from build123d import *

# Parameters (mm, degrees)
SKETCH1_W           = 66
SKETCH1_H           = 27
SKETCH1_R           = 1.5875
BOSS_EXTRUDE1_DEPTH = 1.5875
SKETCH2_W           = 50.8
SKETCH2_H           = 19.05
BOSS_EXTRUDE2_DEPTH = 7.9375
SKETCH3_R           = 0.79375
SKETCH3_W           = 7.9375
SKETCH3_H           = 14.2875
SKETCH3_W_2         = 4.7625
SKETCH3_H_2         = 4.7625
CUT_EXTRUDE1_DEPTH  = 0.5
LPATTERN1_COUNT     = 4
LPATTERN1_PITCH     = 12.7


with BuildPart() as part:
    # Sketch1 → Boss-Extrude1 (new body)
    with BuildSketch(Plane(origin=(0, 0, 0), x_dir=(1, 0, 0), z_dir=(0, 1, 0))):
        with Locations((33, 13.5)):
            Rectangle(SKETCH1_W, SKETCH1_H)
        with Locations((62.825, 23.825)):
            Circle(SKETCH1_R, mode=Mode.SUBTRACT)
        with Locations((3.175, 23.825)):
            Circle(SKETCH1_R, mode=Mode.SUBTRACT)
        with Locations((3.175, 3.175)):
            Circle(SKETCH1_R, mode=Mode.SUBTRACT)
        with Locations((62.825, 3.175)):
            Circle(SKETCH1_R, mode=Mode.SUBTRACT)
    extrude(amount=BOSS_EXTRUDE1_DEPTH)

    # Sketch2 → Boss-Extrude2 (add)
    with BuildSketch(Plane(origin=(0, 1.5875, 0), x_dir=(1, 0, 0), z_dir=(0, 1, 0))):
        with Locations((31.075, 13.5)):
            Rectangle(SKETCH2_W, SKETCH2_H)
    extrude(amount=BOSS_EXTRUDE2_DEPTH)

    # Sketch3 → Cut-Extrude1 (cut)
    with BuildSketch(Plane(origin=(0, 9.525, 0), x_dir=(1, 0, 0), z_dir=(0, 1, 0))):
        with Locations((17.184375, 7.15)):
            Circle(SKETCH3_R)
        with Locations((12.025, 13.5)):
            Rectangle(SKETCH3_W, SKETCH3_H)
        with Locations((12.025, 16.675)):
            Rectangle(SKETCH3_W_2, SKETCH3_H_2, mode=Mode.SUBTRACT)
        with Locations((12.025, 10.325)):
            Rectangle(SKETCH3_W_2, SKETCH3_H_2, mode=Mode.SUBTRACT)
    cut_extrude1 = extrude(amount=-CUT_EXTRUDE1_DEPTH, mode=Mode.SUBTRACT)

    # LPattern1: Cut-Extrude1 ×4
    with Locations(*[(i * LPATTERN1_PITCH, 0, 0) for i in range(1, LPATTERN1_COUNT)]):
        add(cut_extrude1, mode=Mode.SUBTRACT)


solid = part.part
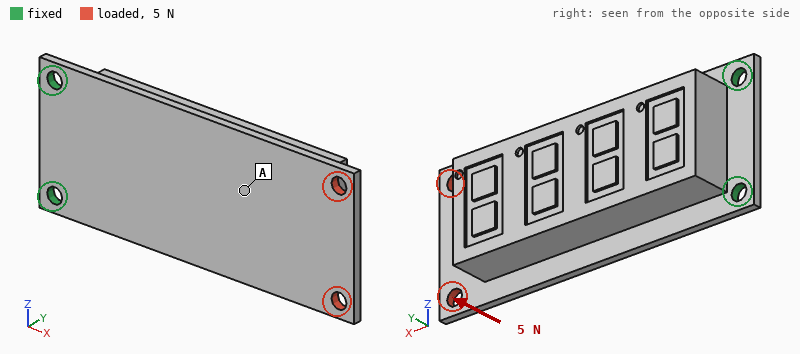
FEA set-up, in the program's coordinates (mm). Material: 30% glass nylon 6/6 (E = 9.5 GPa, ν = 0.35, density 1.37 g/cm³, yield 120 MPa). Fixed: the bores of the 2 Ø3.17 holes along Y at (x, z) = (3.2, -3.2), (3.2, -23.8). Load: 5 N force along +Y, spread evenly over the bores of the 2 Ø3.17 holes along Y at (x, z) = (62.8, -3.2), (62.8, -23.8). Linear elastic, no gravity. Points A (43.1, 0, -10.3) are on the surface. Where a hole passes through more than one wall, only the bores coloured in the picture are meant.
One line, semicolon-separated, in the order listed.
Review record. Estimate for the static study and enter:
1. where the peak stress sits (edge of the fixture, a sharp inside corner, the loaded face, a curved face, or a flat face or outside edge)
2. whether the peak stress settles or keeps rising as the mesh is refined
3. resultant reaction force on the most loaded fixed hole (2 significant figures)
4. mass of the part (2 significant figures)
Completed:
edge of the fixture; keeps rising; 2.8 N; 14 g
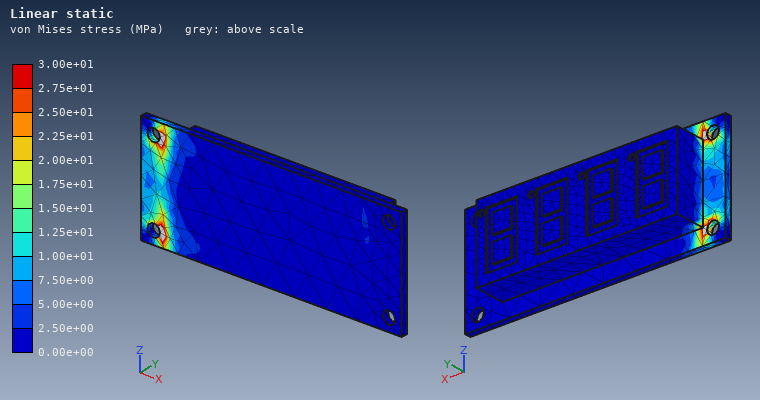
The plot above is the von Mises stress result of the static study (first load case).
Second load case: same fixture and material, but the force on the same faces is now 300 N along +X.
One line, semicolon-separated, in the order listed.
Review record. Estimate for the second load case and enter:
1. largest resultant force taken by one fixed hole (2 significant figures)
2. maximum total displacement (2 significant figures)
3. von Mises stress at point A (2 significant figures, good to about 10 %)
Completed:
150 N; 0.17 mm; 4.4 MPa
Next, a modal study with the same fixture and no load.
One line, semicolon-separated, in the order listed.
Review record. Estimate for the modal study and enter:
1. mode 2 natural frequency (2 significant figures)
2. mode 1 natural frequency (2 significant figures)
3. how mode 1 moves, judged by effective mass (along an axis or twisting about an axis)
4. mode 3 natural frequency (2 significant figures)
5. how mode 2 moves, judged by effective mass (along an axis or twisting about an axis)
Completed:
2000 Hz; 210 Hz; along Y; 3700 Hz; along Z
